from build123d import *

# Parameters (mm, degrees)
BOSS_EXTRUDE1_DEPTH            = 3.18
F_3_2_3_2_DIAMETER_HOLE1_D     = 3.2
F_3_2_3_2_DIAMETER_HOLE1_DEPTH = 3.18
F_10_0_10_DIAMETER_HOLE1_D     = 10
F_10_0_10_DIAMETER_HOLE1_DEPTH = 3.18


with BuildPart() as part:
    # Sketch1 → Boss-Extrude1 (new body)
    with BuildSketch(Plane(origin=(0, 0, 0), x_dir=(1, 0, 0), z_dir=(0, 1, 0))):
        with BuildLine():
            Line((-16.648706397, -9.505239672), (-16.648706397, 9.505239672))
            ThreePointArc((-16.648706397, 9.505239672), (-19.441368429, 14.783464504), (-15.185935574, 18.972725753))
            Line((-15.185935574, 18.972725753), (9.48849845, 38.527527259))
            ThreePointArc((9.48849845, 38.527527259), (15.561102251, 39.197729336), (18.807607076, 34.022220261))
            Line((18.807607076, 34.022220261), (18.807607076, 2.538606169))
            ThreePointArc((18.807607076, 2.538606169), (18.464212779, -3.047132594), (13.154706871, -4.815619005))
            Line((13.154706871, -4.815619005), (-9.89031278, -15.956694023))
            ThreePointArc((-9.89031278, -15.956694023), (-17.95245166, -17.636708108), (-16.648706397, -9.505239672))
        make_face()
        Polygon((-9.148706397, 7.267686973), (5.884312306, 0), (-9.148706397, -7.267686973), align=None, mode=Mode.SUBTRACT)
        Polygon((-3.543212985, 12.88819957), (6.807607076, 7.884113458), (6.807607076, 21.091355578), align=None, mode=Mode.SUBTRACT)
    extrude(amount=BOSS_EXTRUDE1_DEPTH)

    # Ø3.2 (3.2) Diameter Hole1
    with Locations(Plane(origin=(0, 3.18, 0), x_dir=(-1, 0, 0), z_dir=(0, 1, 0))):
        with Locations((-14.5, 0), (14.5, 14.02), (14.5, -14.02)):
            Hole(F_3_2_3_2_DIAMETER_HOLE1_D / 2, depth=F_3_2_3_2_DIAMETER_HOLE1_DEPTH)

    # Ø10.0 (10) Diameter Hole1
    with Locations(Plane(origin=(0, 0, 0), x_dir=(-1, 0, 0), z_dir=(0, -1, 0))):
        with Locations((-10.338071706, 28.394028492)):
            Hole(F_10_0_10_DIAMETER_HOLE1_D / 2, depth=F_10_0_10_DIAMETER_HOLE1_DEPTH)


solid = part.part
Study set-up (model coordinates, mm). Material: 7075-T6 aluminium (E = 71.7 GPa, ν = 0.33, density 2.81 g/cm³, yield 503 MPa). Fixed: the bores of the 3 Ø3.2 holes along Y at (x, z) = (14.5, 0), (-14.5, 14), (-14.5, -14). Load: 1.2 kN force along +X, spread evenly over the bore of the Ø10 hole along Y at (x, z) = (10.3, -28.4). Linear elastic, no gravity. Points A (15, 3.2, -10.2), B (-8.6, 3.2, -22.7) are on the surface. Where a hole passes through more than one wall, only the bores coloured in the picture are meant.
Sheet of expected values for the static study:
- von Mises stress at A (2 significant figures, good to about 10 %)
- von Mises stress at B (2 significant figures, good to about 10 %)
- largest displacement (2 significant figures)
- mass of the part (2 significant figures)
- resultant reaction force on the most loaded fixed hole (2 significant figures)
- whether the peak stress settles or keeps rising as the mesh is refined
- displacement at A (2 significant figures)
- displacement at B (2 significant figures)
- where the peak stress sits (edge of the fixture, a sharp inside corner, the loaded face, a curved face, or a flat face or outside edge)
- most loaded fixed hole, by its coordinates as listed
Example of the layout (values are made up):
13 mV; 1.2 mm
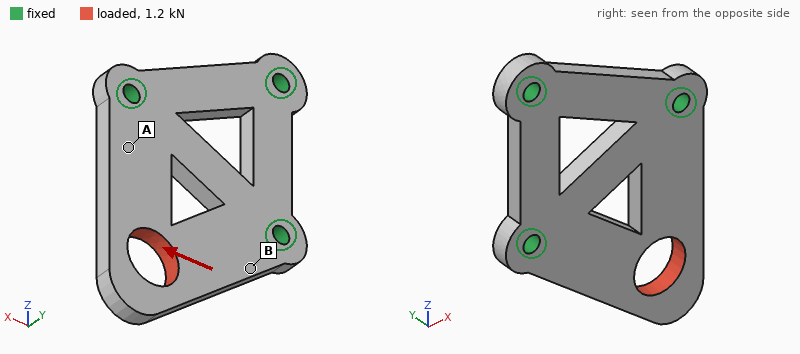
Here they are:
23 MPa; 44 MPa; 38 µm; 11 g; 1.2 kN; keeps rising; 6.7 µm; 8.7 µm; a sharp inside corner; (-14.5, -14)
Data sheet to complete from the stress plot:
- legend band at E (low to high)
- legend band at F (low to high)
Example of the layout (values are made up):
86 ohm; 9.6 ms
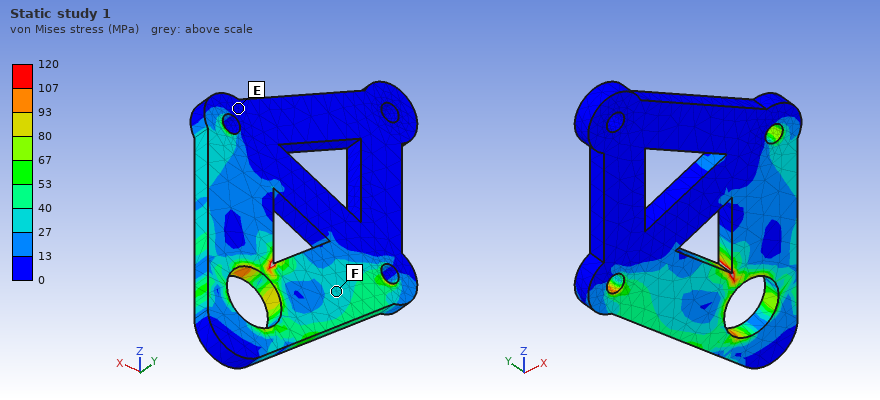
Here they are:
0 to 13 MPa; 27 to 40 MPa
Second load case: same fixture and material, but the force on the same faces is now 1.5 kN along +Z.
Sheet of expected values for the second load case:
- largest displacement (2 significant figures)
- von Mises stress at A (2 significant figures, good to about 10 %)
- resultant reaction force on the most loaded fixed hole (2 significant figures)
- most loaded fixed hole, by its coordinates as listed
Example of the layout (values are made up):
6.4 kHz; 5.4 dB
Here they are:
26 µm; 39 MPa; 1.2 kN; (14.5, 0)
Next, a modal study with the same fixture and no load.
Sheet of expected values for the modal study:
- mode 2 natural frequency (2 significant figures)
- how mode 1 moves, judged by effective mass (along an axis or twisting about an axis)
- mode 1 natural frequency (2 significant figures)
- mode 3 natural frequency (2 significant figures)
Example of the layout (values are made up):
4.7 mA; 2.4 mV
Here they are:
10 kHz; along Y; 2800 Hz; 11 kHz
